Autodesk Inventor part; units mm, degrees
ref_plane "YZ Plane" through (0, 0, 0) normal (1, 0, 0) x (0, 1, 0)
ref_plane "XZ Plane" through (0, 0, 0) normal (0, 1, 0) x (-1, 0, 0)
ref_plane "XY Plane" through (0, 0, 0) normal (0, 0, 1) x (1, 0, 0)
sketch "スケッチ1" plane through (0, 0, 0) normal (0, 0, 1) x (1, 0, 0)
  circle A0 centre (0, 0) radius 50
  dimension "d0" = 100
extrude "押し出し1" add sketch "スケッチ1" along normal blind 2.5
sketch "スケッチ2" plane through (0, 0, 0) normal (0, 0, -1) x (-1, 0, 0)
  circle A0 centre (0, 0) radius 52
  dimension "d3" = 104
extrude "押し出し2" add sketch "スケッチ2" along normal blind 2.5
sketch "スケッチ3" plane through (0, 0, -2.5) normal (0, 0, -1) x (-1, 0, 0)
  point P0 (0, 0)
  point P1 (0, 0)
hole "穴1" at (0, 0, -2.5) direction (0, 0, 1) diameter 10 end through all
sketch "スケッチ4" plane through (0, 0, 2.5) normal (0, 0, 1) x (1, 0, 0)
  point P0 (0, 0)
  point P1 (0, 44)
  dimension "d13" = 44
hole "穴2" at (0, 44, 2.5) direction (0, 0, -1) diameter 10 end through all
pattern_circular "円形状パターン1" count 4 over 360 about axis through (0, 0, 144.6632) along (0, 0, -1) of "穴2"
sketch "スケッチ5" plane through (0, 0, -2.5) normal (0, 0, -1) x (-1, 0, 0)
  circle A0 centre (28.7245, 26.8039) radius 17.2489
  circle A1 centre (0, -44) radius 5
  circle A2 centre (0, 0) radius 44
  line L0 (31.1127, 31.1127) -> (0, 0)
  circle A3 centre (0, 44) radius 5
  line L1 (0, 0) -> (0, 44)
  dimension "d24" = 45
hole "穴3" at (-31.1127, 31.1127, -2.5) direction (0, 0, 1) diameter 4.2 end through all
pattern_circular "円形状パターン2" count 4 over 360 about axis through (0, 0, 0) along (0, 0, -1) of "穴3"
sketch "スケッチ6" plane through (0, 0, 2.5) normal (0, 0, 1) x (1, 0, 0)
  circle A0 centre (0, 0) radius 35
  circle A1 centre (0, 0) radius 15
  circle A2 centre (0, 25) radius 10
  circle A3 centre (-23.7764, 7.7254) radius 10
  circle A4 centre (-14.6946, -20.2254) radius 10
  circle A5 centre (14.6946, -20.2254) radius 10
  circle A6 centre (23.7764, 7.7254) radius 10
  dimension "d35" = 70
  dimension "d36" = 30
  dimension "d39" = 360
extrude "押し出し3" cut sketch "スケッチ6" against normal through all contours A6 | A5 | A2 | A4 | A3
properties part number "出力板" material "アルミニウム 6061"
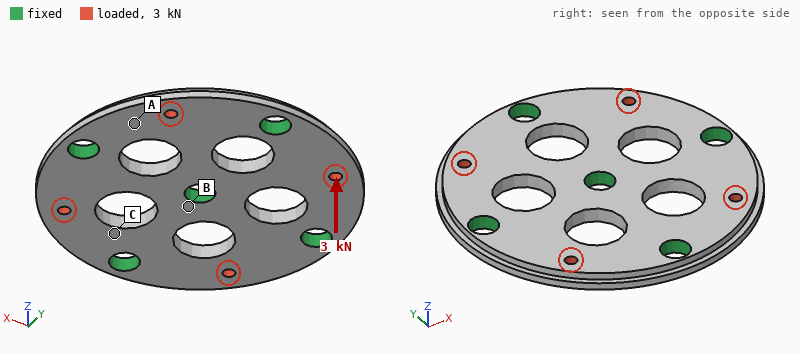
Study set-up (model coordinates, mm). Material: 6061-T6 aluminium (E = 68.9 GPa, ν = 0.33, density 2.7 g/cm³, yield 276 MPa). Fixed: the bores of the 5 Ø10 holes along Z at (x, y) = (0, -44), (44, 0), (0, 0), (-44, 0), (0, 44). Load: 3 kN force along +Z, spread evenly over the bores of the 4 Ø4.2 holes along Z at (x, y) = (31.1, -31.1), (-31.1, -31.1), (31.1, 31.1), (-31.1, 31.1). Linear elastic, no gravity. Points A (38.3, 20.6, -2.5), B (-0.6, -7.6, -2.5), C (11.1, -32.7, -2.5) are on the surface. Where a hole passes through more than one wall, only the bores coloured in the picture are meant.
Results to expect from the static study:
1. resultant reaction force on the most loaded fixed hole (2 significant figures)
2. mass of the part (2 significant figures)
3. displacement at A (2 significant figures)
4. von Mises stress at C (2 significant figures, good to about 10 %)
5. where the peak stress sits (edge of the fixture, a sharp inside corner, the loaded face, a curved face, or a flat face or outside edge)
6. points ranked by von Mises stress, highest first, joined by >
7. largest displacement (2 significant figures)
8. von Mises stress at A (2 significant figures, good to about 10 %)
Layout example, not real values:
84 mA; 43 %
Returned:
760 N; 83 g; 0.052 mm; 44 MPa; the loaded face; C > A > B; 0.12 mm; 25 MPa
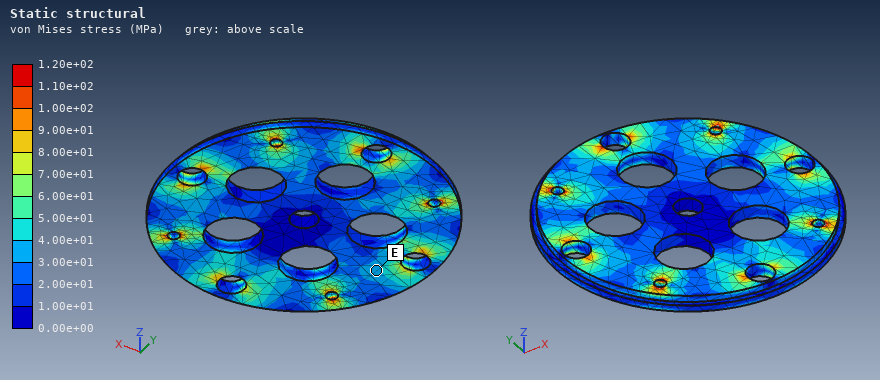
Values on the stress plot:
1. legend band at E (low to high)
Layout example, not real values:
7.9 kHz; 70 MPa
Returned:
3.00e+01 to 4.00e+01 MPa
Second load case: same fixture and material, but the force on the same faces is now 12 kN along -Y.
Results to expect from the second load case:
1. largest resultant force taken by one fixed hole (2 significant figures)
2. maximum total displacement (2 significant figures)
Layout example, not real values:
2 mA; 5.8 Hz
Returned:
3.8 kN; 18 µm
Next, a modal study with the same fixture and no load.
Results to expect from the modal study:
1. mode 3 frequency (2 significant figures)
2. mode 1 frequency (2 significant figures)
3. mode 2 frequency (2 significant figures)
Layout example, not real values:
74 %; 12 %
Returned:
6600 Hz; 6400 Hz; 6500 Hz
